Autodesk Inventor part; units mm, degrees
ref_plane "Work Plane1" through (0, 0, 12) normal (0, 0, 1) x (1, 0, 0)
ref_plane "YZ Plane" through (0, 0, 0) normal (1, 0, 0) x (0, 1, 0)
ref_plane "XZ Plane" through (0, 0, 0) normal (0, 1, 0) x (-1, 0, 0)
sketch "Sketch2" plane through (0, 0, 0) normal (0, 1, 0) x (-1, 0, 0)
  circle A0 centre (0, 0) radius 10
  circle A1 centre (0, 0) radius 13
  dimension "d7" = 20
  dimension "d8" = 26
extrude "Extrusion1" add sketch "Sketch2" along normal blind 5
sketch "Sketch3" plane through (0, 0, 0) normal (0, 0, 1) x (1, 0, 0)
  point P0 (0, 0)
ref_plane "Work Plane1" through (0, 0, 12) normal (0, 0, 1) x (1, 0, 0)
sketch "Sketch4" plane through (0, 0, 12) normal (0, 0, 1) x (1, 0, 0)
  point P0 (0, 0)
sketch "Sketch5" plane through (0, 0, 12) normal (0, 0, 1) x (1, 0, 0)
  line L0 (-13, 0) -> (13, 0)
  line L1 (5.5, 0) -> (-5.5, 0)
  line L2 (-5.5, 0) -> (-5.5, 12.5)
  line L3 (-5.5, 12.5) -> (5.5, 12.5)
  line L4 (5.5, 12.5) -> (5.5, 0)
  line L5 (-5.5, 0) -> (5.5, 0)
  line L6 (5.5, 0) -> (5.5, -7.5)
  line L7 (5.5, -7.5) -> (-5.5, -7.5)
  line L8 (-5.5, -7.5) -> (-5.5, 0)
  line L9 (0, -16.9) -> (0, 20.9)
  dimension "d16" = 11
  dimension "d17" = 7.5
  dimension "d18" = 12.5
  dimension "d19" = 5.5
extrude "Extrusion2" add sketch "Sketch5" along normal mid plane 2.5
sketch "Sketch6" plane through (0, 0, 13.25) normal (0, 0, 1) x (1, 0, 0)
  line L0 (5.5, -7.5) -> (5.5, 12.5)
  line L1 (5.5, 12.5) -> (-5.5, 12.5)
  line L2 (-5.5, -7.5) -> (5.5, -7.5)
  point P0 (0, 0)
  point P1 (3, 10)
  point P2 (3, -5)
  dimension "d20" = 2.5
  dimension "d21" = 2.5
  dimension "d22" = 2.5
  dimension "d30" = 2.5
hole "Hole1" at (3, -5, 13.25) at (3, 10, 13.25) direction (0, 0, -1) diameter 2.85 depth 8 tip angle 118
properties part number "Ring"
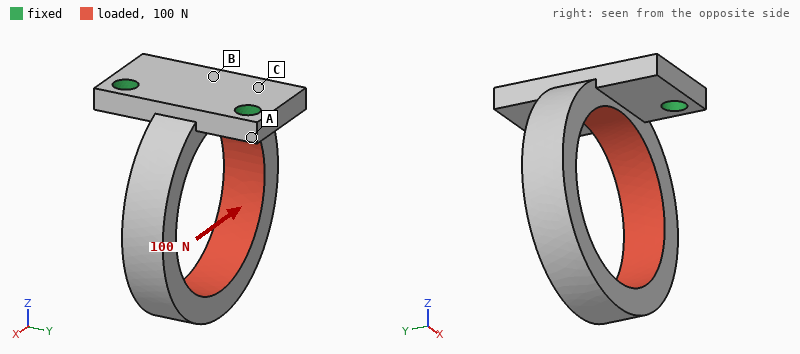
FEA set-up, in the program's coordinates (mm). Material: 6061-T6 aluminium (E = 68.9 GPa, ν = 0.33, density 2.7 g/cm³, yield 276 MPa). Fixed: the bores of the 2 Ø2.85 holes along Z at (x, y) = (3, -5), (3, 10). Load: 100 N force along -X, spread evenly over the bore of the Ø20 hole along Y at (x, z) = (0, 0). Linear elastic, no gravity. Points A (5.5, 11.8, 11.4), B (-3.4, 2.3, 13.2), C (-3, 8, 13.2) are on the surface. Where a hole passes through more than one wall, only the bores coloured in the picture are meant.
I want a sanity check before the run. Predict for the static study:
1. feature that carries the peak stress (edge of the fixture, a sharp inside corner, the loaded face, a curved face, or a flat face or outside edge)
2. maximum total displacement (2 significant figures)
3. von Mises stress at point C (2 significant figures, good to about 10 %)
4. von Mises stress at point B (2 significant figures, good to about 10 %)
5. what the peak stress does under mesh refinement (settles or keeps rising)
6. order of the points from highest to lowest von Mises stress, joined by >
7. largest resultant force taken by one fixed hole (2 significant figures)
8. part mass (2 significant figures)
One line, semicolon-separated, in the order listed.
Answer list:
edge of the fixture; 0.12 mm; 18 MPa; 32 MPa; keeps rising; B > C > A; 65 N; 4.1 g
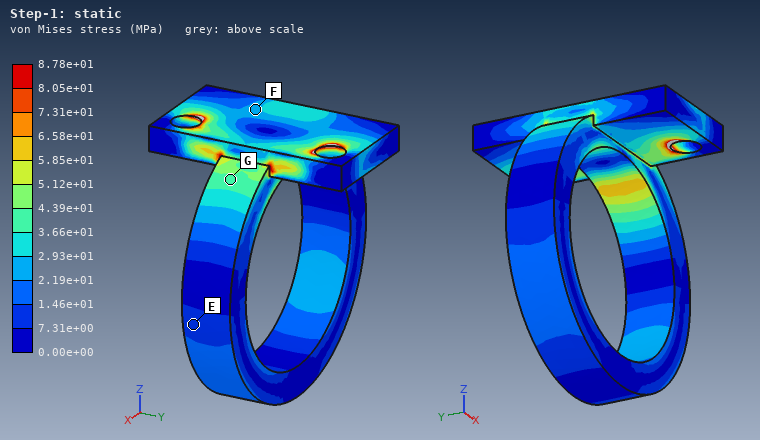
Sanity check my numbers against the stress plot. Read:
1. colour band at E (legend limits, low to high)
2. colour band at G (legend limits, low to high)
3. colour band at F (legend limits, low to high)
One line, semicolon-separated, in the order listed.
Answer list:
7.31e+00 to 1.46e+01 MPa; 3.66e+01 to 4.39e+01 MPa; 2.19e+01 to 2.93e+01 MPa
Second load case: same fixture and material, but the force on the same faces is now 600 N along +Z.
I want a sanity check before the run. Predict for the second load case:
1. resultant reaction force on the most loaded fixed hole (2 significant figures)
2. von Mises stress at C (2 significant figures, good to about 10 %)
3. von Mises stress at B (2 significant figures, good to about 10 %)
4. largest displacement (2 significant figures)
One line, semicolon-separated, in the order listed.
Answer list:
320 N; 42 MPa; 75 MPa; 0.12 mm
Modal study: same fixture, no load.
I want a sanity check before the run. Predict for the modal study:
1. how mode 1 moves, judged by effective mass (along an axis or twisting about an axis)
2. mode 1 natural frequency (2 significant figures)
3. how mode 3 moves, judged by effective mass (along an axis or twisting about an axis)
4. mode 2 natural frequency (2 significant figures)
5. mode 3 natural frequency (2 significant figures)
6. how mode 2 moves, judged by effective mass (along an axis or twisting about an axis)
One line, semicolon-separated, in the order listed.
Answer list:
along X; 2800 Hz; twisting about Z; 3300 Hz; 8700 Hz; along Y
